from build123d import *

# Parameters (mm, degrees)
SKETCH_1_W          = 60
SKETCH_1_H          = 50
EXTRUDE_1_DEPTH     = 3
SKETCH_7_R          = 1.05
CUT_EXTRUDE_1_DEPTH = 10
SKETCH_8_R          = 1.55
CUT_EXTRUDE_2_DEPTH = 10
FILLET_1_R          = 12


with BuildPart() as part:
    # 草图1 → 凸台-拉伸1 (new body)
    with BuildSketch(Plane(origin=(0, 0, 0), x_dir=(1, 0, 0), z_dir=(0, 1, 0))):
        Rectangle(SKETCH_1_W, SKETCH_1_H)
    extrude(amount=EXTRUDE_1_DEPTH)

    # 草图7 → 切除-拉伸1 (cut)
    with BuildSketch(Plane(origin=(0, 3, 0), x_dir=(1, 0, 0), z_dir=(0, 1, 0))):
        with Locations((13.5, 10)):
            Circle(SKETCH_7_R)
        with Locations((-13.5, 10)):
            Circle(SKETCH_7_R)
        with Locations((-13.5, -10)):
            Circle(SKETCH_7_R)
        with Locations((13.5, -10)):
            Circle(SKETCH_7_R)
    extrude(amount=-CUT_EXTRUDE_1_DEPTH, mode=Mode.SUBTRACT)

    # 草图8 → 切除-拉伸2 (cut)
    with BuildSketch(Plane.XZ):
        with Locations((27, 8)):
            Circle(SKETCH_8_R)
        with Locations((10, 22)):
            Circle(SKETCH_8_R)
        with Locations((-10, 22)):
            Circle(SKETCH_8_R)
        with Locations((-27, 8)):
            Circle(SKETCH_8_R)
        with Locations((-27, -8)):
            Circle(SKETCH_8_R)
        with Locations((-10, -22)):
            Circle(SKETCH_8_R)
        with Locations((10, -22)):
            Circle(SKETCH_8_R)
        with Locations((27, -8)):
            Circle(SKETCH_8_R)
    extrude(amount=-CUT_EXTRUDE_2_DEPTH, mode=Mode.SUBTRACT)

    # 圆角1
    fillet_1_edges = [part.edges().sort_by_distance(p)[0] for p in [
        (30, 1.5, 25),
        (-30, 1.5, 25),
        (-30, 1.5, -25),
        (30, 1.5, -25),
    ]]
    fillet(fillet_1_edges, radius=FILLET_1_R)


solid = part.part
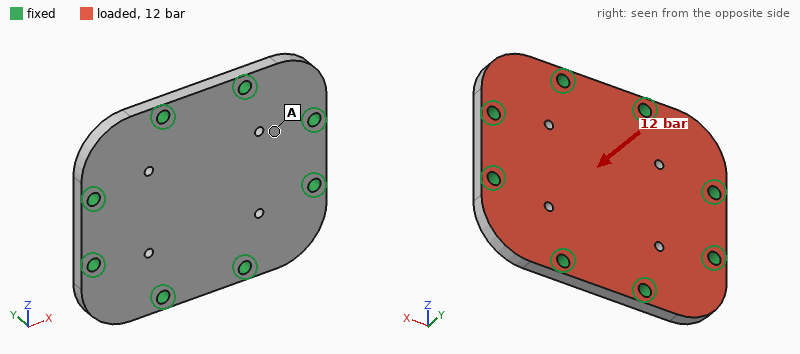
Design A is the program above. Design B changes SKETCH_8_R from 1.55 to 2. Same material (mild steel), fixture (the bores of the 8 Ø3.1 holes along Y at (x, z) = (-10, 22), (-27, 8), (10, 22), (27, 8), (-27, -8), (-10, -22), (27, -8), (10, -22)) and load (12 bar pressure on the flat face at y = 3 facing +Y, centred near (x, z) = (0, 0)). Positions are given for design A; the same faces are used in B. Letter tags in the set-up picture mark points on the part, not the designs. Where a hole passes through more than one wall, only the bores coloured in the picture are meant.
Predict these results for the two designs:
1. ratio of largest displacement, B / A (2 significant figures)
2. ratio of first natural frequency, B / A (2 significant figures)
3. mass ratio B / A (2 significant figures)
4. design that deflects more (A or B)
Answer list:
0.90
1.1
0.99
A
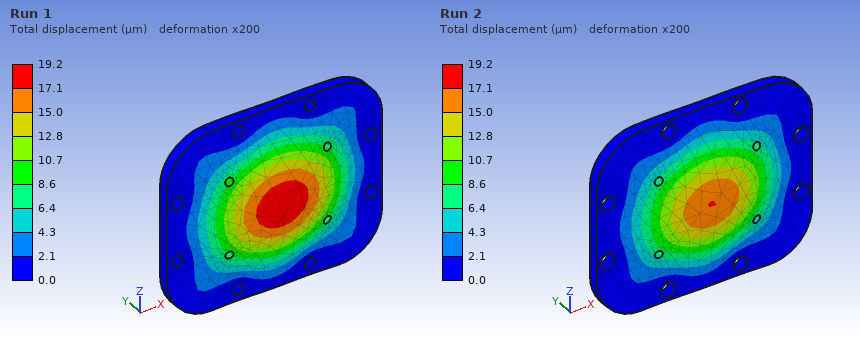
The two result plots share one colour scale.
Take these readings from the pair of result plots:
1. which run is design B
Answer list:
Run 2
